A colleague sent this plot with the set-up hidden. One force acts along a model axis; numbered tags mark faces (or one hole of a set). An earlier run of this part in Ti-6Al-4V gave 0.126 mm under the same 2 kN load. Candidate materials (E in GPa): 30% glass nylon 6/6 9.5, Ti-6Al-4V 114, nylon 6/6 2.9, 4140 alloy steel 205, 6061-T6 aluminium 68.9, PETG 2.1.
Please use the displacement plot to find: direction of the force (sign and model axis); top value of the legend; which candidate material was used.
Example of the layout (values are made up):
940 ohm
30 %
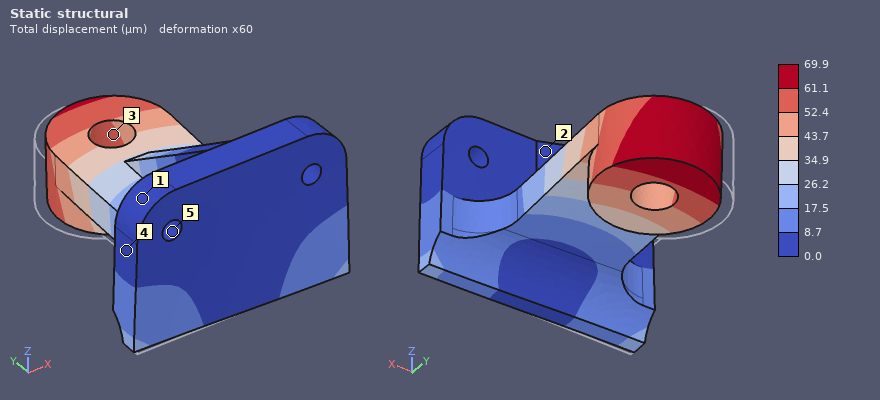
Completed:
+X
69.9 µm
4140 alloy steel
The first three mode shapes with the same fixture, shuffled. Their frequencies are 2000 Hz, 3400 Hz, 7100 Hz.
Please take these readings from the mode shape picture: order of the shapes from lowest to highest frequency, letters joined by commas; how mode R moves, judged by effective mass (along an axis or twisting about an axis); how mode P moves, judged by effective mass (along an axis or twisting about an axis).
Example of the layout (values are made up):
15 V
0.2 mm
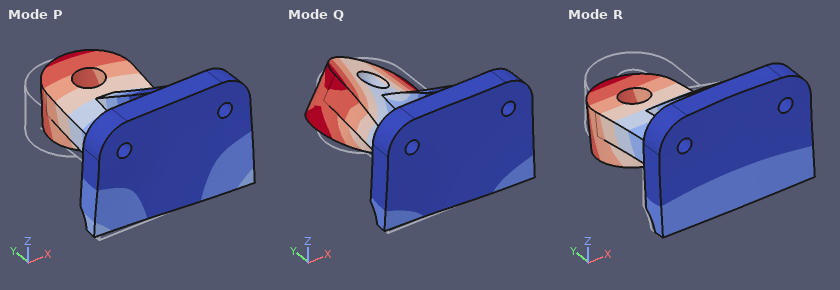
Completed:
R, P, Q
along Z
along X
